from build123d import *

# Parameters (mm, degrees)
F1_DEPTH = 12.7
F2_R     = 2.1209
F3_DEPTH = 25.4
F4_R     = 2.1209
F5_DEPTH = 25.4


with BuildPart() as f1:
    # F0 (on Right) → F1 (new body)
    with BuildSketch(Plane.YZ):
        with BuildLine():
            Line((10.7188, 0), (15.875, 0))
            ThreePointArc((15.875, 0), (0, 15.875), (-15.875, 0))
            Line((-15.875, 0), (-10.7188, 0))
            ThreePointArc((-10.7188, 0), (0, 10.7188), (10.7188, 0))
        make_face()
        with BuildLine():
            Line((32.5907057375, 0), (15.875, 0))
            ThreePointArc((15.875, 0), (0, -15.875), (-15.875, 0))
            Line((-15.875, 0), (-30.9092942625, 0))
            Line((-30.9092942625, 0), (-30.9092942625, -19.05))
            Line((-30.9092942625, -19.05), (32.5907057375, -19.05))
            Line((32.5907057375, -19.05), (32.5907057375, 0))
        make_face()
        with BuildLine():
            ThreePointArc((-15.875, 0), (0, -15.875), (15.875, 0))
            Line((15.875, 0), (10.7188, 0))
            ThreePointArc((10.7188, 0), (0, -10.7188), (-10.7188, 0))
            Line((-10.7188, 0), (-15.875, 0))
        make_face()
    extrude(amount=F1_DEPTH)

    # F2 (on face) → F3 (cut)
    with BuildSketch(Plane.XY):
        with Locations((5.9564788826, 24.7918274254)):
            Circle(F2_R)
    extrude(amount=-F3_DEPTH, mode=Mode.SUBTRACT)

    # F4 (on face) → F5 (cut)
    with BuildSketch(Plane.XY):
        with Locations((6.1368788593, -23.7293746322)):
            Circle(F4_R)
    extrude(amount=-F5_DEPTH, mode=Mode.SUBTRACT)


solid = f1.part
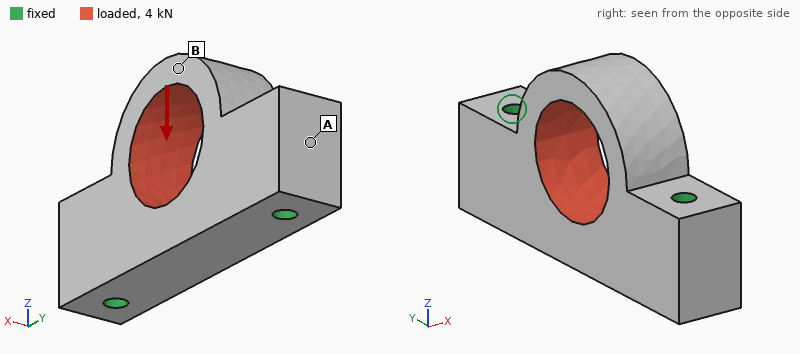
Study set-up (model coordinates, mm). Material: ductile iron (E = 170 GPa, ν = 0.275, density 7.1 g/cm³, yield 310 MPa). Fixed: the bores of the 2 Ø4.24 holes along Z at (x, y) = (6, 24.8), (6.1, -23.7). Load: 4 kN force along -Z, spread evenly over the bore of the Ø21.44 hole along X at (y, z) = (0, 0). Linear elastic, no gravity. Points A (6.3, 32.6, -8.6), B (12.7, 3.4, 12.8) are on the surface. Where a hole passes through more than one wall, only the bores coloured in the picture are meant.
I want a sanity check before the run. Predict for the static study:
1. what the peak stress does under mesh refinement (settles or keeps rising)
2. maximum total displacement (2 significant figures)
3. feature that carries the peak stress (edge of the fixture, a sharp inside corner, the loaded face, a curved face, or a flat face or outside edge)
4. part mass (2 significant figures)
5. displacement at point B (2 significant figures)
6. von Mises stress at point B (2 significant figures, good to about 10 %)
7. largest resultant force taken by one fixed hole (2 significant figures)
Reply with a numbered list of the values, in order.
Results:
1. keeps rising
2. 4.0 µm
3. edge of the fixture
4. 110 g
5. 3.8 µm
6. 11 MPa
7. 2.0 kN
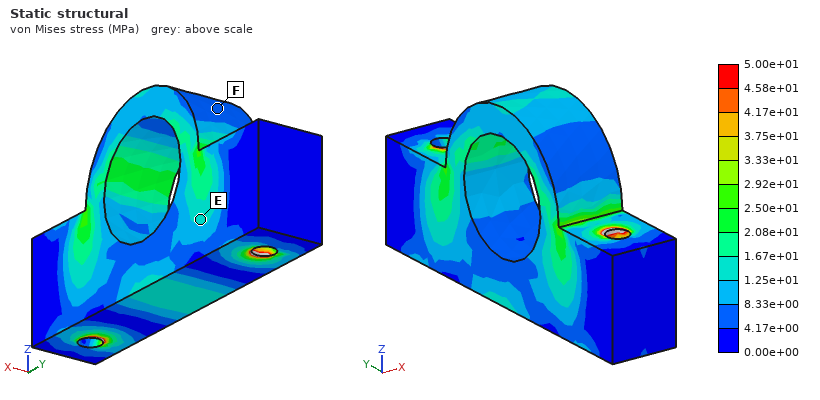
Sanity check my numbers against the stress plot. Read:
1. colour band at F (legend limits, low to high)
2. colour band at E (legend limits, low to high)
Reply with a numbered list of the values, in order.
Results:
1. 4.17e+00 to 8.33e+00 MPa
2. 1.25e+01 to 1.67e+01 MPa
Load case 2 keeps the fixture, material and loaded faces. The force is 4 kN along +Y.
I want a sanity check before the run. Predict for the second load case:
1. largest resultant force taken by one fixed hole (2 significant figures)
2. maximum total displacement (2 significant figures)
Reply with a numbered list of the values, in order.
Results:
1. 2.1 kN
2. 9.4 µm
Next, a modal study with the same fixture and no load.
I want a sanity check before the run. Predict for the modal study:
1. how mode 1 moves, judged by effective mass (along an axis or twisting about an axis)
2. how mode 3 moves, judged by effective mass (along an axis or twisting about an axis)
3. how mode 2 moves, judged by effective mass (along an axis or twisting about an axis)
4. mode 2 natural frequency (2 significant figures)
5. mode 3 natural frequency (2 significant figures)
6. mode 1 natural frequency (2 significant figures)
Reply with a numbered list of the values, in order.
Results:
1. along X
2. along X
3. along Y
4. 18 kHz
5. 19 kHz
6. 11 kHz
